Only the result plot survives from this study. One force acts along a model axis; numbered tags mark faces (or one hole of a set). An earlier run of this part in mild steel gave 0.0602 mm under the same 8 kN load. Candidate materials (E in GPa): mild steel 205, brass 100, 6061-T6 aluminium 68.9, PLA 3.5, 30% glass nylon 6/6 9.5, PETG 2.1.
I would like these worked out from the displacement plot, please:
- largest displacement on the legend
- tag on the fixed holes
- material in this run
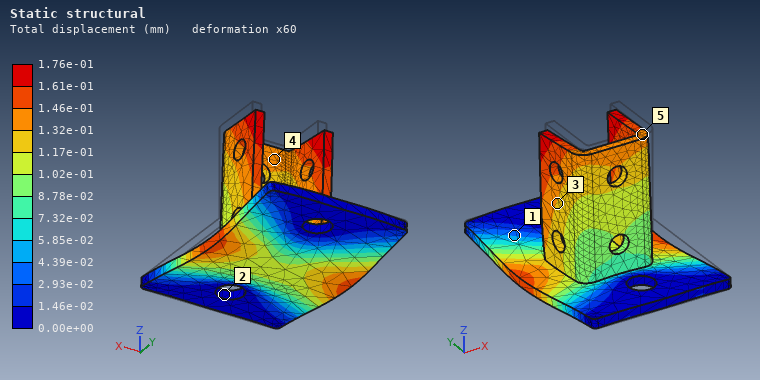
1.76e-01 mm
2
6061-T6 aluminium
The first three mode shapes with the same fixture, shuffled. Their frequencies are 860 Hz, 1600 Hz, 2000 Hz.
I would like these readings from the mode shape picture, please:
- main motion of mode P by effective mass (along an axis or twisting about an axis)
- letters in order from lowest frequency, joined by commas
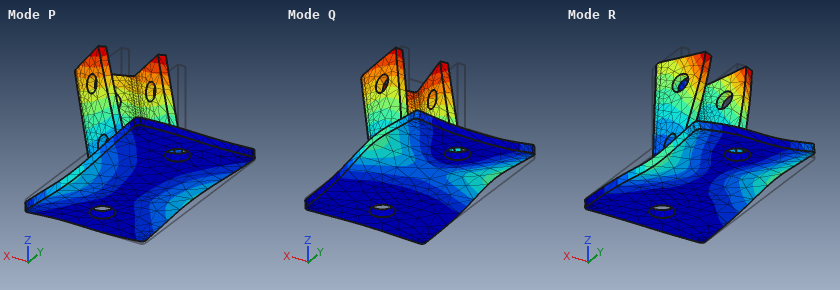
along X
P, Q, R
